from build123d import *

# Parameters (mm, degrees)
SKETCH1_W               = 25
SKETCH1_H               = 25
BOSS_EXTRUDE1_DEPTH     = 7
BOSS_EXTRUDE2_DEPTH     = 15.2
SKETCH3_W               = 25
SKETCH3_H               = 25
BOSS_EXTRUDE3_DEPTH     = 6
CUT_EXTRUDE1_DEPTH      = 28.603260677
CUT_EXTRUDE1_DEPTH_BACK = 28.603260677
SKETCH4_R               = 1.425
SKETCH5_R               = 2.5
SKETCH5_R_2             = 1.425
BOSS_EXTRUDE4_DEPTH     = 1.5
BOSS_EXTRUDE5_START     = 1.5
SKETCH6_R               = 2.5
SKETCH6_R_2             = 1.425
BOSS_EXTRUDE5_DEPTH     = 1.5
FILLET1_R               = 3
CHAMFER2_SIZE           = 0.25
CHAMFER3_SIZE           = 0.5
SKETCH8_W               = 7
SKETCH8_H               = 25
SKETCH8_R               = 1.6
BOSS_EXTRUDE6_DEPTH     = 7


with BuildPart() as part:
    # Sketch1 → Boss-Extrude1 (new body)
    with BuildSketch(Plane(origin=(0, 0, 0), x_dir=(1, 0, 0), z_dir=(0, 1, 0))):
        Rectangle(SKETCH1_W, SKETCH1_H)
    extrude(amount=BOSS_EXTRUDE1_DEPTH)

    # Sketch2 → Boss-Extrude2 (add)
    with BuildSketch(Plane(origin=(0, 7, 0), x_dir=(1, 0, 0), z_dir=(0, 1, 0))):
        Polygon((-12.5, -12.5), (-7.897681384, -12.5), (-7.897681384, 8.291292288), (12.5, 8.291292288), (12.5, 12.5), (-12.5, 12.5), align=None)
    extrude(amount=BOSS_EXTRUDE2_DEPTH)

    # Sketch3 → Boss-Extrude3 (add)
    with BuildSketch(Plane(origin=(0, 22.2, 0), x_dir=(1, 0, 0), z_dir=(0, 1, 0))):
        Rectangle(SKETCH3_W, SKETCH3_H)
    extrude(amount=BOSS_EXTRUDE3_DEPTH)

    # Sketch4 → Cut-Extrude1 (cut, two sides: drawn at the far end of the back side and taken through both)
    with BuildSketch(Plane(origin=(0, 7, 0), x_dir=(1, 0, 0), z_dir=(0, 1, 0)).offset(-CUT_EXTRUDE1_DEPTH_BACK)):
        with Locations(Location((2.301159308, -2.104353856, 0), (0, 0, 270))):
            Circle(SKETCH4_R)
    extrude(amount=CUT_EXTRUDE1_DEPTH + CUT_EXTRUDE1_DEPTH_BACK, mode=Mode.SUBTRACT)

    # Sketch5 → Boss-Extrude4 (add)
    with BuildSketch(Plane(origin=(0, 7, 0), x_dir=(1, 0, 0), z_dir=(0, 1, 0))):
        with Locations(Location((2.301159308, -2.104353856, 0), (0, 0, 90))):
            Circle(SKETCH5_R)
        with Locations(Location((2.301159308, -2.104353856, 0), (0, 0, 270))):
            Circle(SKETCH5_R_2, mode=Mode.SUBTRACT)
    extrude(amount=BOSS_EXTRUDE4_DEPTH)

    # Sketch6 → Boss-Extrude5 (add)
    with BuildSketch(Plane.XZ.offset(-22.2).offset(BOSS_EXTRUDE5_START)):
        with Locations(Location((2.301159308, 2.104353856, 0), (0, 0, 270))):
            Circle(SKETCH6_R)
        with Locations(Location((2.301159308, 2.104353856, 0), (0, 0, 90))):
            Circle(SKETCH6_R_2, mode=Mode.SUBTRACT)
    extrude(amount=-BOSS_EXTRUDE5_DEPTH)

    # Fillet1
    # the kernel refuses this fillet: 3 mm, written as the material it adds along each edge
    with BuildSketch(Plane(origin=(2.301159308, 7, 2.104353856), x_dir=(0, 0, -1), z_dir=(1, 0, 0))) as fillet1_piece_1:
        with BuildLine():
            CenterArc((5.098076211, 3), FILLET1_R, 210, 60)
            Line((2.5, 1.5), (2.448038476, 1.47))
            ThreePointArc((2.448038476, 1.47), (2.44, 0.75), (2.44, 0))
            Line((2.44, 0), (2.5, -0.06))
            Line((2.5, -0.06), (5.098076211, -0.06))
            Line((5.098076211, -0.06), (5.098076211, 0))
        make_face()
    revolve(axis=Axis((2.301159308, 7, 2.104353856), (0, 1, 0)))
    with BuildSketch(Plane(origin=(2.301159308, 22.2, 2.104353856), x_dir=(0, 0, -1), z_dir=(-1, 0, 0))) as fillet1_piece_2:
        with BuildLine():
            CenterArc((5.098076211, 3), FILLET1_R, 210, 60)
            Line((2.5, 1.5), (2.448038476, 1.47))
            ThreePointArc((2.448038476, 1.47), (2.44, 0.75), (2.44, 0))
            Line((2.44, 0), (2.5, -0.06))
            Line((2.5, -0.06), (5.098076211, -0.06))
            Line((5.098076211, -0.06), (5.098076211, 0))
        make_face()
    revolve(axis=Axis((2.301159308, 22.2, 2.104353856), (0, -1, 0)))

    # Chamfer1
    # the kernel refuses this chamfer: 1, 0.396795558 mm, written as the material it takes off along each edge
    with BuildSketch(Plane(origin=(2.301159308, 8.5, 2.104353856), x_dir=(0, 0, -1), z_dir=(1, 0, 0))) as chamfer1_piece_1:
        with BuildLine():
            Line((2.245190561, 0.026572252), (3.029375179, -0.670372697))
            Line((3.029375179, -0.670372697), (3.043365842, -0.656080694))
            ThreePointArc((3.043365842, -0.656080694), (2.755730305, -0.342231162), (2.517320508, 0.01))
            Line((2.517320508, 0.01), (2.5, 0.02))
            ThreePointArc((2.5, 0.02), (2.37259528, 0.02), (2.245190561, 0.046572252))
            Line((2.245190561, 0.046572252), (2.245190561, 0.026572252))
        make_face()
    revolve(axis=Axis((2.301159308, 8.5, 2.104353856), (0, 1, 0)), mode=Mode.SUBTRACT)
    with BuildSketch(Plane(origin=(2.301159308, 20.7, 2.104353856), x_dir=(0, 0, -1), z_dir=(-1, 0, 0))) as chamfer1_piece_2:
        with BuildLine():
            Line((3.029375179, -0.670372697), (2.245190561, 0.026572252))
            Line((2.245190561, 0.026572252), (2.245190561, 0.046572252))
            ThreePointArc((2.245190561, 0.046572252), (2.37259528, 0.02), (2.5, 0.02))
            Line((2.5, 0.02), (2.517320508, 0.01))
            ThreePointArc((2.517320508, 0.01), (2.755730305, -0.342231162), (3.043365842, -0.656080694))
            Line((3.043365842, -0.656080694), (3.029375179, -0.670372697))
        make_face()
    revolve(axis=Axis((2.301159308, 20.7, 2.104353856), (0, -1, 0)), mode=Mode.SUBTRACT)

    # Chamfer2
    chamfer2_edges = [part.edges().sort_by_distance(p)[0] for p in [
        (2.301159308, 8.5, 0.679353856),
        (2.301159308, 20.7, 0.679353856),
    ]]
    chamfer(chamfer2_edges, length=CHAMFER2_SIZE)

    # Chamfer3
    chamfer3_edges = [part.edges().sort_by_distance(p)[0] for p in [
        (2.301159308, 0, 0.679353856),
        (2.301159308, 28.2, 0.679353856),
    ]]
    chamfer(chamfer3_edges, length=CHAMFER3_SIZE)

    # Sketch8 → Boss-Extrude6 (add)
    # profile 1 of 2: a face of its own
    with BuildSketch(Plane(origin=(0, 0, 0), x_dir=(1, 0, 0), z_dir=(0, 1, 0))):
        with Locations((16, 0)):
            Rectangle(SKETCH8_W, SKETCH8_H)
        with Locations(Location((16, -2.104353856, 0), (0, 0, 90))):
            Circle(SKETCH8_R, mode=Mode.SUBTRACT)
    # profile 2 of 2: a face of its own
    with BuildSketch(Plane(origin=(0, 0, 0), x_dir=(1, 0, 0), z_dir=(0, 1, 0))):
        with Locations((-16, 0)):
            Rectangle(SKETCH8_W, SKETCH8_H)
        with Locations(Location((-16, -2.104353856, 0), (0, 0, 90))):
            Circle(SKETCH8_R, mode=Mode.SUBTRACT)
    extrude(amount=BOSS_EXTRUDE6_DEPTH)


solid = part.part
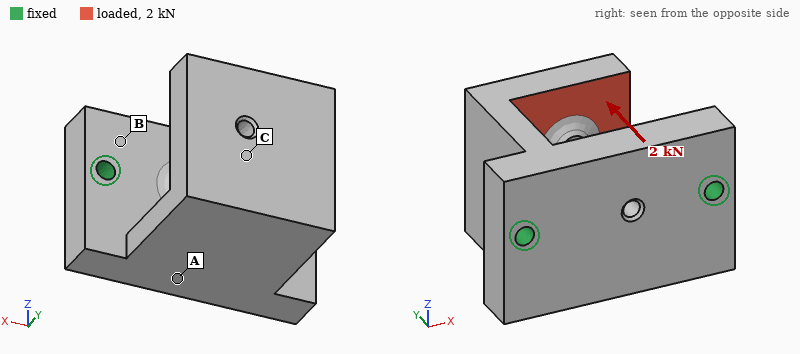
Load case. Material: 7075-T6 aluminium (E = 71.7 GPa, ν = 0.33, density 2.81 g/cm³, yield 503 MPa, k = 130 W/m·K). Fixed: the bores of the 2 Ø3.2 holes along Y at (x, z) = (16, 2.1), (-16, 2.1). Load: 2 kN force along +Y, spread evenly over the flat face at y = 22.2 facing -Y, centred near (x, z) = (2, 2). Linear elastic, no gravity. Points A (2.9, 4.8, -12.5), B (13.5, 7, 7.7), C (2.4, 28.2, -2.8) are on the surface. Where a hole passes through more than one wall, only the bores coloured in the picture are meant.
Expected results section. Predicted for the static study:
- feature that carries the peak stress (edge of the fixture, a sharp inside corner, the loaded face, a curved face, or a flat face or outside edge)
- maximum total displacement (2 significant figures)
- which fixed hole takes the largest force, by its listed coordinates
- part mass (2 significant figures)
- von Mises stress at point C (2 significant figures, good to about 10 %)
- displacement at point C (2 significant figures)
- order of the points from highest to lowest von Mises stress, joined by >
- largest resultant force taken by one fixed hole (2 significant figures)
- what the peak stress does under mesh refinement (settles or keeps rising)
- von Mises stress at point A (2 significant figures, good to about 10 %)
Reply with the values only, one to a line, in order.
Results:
edge of the fixture
0.17 mm
(16, 2.1)
38 g
66 MPa
0.070 mm
C > A > B
1.1 kN
keeps rising
44 MPa
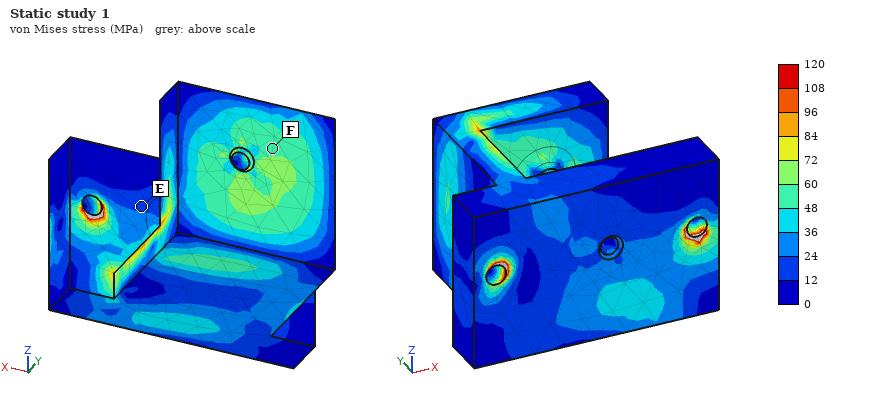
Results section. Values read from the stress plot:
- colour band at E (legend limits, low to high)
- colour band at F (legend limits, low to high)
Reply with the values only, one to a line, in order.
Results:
12 to 24 MPa
48 to 60 MPa
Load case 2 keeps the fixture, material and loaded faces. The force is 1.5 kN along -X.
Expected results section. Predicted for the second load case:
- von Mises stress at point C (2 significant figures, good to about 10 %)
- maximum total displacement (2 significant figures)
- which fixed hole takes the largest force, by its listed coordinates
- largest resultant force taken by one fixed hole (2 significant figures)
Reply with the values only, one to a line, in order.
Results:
10 MPa
0.11 mm
(-16, 2.1)
1.3 kN
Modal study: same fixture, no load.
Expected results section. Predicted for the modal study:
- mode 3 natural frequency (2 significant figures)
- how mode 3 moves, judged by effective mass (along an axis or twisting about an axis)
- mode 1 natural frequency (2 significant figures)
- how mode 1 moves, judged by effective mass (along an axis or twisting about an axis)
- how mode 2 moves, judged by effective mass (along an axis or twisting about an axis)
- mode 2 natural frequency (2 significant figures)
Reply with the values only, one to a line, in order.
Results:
10 kHz
along Y
4900 Hz
along Z
along X
5900 Hz
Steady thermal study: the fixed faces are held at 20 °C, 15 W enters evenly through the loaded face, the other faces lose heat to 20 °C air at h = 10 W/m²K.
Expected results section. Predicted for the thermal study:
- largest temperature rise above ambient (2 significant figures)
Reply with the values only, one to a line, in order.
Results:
22 K
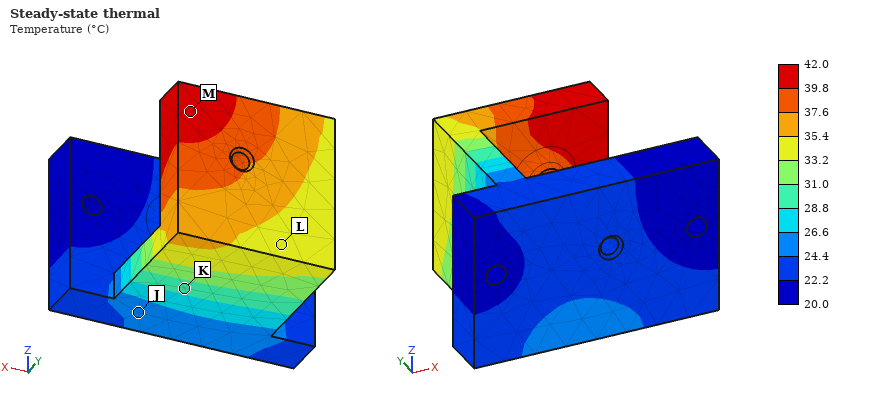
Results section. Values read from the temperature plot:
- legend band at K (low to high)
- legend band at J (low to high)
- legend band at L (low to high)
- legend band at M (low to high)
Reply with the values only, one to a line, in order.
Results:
28.8 to 31.0 °C
24.4 to 26.6 °C
33.2 to 35.4 °C
39.8 to 42.0 °C
